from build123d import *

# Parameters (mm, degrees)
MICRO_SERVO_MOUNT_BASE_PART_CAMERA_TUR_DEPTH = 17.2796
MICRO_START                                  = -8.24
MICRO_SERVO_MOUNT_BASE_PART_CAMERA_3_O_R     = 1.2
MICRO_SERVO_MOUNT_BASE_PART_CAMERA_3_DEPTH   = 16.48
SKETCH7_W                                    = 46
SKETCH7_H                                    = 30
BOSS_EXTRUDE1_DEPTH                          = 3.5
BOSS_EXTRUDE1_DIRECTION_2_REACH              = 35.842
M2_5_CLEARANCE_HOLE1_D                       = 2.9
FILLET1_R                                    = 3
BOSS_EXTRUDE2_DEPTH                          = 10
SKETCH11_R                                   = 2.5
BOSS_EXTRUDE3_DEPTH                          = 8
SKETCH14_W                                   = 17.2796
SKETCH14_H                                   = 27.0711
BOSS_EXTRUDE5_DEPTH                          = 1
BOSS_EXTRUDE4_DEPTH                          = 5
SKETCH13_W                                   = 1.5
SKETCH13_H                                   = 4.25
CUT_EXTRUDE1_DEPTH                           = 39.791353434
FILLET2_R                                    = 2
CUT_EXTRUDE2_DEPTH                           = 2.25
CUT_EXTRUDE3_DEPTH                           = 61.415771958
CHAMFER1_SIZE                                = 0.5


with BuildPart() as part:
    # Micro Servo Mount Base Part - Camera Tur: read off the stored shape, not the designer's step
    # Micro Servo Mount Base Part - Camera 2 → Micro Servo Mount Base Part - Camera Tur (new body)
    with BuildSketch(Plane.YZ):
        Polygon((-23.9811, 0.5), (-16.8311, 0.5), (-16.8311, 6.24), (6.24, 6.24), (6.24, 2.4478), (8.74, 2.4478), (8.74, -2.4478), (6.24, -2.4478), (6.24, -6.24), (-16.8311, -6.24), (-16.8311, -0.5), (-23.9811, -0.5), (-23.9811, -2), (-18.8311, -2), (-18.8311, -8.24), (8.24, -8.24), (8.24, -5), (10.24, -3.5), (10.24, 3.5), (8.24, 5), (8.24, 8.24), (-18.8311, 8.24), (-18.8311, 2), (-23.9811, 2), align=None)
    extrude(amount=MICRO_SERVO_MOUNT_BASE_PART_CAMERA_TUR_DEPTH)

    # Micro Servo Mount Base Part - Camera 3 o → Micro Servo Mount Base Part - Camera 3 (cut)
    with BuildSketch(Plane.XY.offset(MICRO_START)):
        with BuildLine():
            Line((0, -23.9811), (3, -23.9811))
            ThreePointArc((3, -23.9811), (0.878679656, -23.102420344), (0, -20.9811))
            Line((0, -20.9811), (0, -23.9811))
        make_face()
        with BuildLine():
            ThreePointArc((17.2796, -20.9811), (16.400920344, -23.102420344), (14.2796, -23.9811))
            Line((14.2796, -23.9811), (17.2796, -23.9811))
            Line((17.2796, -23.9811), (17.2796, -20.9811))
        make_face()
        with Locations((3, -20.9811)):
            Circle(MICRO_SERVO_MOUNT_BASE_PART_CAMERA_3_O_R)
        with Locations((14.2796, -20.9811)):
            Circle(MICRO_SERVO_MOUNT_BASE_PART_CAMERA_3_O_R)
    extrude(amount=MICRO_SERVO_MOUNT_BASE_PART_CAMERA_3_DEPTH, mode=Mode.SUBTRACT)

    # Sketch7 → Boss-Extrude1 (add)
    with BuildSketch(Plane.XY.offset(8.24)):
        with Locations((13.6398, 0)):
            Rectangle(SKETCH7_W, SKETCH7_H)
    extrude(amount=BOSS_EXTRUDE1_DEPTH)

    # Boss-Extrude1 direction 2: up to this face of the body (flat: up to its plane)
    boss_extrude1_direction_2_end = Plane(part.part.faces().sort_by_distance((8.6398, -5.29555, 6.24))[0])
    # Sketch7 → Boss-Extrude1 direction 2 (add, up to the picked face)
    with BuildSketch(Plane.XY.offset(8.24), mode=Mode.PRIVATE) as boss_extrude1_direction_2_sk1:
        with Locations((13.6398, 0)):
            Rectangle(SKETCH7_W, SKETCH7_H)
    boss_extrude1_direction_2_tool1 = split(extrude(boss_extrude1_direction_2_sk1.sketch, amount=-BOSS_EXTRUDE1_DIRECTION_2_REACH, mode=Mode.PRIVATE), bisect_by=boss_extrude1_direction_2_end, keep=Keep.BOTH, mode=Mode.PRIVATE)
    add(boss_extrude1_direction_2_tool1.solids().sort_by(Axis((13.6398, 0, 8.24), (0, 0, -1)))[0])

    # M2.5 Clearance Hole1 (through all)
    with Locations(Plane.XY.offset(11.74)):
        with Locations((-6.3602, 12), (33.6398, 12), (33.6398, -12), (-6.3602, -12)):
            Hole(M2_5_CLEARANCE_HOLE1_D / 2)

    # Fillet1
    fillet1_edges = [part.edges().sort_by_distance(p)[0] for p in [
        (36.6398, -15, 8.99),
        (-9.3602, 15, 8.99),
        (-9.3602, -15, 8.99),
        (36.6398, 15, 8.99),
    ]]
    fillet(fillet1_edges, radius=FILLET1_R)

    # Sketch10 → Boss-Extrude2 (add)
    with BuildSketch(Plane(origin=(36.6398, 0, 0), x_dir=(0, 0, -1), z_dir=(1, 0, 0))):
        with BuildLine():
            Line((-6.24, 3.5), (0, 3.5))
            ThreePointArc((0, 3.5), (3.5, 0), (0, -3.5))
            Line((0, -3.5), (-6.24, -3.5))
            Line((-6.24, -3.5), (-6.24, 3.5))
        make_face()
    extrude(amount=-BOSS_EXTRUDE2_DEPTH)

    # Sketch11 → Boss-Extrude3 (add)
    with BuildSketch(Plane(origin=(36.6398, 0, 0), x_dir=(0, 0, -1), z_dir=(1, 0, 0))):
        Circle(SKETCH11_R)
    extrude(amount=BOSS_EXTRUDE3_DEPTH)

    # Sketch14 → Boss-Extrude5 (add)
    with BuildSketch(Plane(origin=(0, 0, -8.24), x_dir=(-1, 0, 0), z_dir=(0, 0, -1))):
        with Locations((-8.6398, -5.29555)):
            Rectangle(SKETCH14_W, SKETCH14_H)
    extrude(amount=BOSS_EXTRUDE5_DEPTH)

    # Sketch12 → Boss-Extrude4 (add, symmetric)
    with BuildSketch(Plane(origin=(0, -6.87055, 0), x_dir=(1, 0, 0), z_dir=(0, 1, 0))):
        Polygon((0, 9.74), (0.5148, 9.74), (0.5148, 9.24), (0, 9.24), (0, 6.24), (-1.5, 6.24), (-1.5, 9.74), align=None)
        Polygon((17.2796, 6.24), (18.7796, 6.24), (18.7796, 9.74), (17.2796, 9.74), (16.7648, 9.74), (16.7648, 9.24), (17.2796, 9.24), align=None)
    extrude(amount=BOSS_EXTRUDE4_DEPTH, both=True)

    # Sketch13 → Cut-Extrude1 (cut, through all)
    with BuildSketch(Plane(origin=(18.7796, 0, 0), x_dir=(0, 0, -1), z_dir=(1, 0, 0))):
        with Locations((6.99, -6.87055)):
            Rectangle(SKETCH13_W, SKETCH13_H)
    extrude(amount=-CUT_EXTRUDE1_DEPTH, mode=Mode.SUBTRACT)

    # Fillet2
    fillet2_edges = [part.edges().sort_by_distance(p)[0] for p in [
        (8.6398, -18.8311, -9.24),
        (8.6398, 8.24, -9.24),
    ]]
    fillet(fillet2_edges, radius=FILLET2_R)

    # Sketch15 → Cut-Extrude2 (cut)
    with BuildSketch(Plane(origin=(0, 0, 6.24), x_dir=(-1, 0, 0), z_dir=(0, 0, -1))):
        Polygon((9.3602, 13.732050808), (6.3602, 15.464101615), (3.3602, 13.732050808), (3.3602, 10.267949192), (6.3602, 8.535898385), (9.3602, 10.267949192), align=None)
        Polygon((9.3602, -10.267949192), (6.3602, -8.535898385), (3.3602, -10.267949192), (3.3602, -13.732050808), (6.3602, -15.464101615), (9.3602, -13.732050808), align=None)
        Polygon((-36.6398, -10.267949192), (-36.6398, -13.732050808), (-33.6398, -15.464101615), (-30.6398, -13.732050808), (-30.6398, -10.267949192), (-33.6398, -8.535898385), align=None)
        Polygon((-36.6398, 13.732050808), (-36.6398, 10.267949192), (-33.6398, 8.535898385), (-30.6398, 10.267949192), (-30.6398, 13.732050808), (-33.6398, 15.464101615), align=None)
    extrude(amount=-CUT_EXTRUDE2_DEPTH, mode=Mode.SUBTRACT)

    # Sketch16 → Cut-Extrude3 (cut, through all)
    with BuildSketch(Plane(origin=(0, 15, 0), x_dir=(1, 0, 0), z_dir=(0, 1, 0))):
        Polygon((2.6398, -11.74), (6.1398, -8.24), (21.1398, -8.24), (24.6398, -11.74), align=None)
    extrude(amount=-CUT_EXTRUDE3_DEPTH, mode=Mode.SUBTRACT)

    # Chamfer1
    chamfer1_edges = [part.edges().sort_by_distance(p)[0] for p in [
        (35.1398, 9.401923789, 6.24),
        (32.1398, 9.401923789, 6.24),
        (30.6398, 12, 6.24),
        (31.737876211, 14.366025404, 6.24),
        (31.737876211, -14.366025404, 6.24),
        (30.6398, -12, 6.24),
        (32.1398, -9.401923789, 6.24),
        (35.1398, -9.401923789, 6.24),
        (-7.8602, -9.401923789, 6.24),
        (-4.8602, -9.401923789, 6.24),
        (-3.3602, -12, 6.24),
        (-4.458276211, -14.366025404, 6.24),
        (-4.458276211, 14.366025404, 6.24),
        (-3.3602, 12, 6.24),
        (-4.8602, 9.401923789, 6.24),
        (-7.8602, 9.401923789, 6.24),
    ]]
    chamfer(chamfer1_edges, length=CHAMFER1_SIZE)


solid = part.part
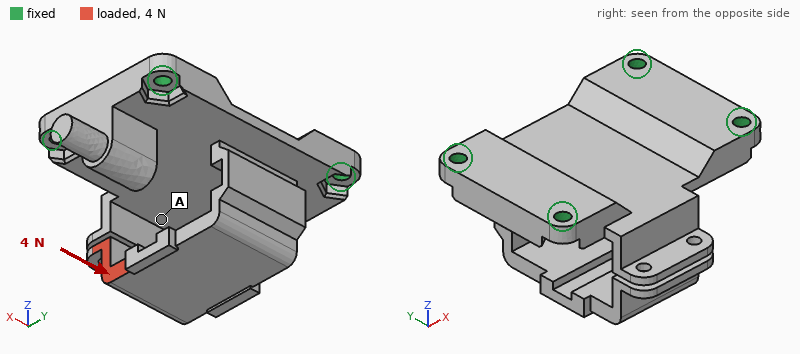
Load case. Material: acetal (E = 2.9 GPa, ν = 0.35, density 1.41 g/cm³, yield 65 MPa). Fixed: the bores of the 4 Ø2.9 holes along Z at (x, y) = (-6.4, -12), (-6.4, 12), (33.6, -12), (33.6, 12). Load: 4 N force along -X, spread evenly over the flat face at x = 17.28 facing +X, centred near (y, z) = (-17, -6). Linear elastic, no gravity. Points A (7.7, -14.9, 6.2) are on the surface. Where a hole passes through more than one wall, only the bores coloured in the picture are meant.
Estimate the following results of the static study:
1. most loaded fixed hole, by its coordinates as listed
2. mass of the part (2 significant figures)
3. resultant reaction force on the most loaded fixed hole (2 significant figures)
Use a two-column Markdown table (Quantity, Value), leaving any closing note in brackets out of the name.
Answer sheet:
| Quantity | Value |
|---|---|
| most loaded fixed hole, by its coordinates as listed | (33.6, 12) |
| mass of the part | 12 g |
| resultant reaction force on the most loaded fixed hole | 5.8 N |
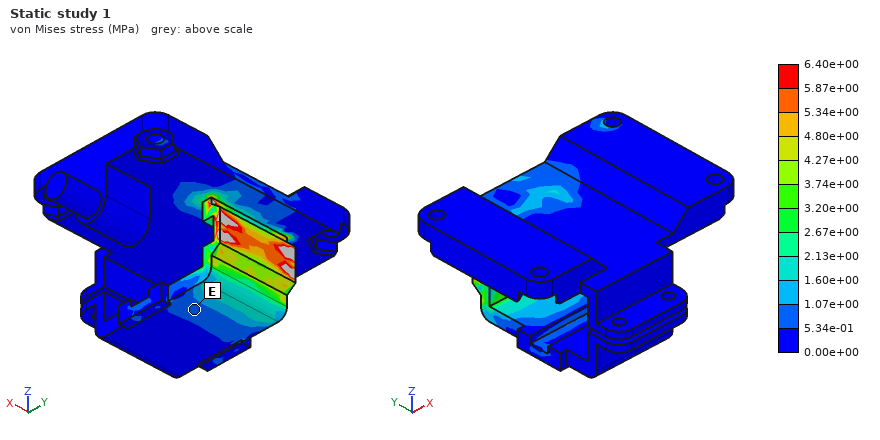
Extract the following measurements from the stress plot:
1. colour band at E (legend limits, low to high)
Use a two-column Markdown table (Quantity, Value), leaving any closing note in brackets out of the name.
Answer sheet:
| Quantity | Value |
|---|---|
| colour band at E | 5.34e-01 to 1.07e+00 MPa |
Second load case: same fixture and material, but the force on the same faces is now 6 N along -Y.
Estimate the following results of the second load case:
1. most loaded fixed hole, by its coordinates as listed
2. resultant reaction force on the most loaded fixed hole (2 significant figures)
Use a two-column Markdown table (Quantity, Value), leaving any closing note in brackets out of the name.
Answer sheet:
| Quantity | Value |
|---|---|
| most loaded fixed hole, by its coordinates as listed | (-6.4, -12) |
| resultant reaction force on the most loaded fixed hole | 5.6 N |
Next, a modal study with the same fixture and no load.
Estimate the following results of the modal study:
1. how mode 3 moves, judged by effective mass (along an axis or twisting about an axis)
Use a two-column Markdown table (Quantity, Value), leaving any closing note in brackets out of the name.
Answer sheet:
| Quantity | Value |
|---|---|
| how mode 3 moves, judged by effective mass | along Y |
